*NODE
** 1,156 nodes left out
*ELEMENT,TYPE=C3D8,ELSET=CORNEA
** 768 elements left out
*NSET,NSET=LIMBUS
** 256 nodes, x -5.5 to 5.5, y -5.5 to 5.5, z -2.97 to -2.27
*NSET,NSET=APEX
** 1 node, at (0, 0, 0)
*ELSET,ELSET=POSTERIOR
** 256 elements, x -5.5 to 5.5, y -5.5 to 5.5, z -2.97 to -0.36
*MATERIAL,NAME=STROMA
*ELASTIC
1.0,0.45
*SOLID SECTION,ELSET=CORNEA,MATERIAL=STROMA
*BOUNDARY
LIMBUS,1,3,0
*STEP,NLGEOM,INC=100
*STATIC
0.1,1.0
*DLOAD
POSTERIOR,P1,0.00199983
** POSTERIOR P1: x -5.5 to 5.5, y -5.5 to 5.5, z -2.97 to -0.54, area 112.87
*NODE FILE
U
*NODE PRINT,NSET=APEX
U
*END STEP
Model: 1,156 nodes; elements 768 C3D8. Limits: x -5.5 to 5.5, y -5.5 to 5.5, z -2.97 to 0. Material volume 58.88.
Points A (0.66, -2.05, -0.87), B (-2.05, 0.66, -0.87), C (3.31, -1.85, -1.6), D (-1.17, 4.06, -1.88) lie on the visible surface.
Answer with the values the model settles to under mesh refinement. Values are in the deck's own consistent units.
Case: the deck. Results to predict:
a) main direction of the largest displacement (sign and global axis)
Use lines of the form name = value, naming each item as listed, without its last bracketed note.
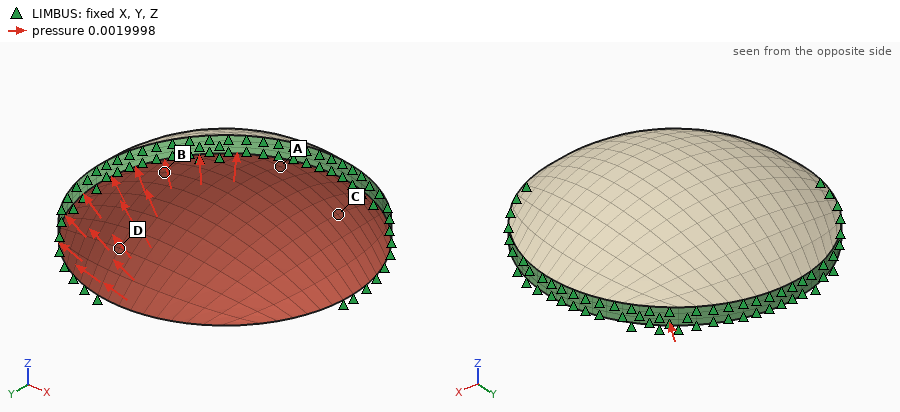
main direction of the largest displacement = +Z
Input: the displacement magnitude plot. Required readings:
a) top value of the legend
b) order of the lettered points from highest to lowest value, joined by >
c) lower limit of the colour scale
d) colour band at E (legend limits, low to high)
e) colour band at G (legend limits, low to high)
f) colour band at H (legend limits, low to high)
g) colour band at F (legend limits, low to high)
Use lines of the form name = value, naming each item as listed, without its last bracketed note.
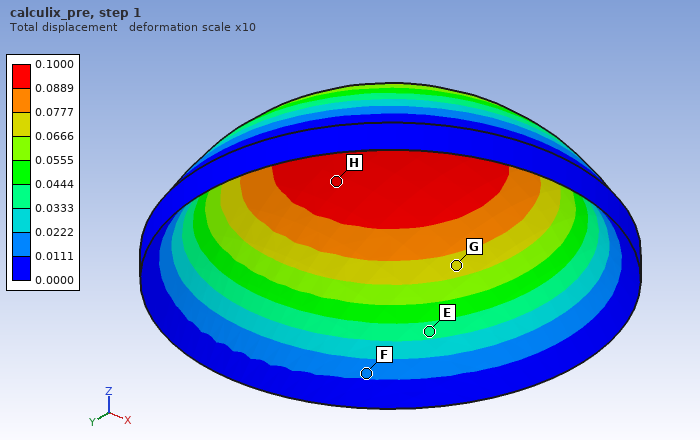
top value of the legend = 0.1000
order of the lettered points from highest to lowest value, joined by > = H > G > E > F
lower limit of the colour scale = 0.0000
colour band at E = 0.0333 to 0.0444
colour band at G = 0.0666 to 0.0777
colour band at H = 0.0889 to 0.1000
colour band at F = 0.0111 to 0.0222
